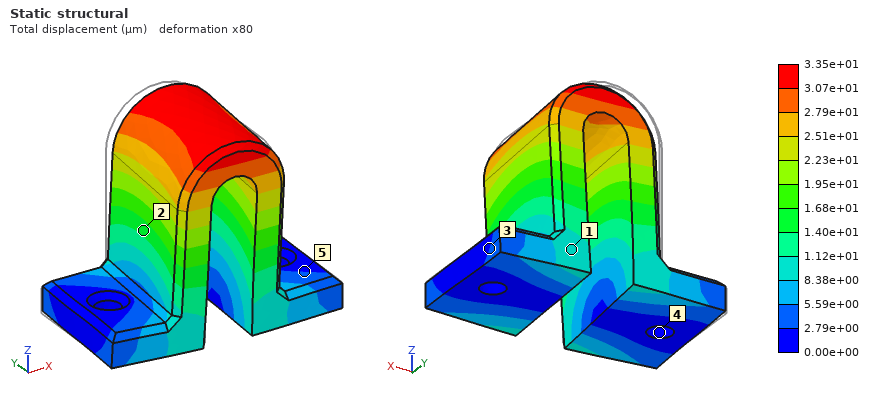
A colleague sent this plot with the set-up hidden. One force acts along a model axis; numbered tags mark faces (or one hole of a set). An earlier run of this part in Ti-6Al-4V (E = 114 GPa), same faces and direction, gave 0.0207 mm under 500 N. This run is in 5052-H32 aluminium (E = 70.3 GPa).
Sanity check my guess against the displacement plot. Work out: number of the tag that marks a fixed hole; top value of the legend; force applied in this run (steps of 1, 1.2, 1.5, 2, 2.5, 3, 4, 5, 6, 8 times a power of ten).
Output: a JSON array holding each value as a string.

["4", "3.35e+01 µm", "500 N"]
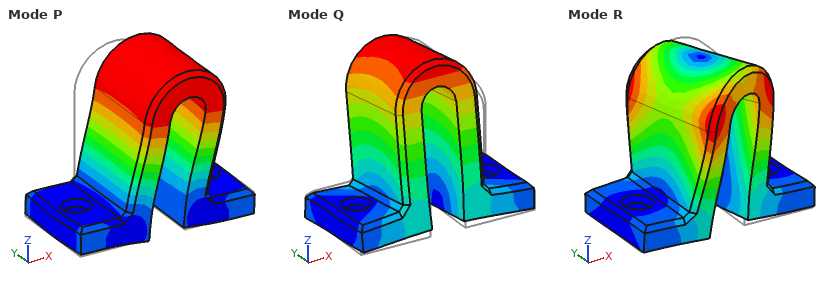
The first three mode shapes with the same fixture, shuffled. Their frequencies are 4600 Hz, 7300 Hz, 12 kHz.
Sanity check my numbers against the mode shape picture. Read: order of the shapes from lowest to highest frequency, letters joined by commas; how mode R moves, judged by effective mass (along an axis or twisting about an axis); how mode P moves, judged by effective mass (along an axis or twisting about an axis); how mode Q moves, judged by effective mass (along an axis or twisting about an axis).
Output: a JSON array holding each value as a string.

["Q, P, R", "twisting about Z", "along X", "along Y"]
